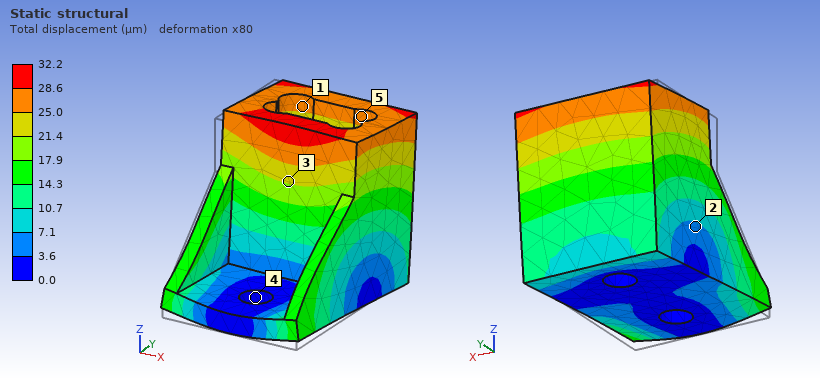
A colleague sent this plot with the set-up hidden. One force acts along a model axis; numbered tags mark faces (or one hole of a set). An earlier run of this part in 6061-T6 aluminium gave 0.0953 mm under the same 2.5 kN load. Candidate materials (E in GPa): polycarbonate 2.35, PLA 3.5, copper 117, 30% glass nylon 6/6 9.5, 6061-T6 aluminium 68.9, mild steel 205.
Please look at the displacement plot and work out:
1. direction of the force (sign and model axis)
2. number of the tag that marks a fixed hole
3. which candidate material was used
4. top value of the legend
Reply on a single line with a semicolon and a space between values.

+Y; 4; mild steel; 32.2 µm
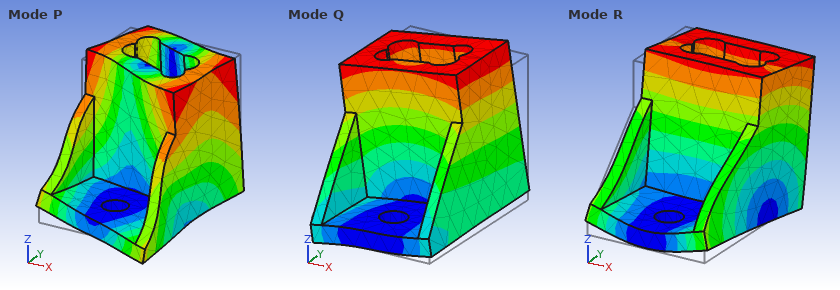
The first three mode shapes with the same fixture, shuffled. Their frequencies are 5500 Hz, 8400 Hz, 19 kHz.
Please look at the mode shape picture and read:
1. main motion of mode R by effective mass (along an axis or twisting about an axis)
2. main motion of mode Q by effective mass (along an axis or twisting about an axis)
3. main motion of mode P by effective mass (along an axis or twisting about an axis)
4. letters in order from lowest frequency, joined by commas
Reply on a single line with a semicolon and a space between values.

along Y; along X; twisting about Z; Q, R, P
